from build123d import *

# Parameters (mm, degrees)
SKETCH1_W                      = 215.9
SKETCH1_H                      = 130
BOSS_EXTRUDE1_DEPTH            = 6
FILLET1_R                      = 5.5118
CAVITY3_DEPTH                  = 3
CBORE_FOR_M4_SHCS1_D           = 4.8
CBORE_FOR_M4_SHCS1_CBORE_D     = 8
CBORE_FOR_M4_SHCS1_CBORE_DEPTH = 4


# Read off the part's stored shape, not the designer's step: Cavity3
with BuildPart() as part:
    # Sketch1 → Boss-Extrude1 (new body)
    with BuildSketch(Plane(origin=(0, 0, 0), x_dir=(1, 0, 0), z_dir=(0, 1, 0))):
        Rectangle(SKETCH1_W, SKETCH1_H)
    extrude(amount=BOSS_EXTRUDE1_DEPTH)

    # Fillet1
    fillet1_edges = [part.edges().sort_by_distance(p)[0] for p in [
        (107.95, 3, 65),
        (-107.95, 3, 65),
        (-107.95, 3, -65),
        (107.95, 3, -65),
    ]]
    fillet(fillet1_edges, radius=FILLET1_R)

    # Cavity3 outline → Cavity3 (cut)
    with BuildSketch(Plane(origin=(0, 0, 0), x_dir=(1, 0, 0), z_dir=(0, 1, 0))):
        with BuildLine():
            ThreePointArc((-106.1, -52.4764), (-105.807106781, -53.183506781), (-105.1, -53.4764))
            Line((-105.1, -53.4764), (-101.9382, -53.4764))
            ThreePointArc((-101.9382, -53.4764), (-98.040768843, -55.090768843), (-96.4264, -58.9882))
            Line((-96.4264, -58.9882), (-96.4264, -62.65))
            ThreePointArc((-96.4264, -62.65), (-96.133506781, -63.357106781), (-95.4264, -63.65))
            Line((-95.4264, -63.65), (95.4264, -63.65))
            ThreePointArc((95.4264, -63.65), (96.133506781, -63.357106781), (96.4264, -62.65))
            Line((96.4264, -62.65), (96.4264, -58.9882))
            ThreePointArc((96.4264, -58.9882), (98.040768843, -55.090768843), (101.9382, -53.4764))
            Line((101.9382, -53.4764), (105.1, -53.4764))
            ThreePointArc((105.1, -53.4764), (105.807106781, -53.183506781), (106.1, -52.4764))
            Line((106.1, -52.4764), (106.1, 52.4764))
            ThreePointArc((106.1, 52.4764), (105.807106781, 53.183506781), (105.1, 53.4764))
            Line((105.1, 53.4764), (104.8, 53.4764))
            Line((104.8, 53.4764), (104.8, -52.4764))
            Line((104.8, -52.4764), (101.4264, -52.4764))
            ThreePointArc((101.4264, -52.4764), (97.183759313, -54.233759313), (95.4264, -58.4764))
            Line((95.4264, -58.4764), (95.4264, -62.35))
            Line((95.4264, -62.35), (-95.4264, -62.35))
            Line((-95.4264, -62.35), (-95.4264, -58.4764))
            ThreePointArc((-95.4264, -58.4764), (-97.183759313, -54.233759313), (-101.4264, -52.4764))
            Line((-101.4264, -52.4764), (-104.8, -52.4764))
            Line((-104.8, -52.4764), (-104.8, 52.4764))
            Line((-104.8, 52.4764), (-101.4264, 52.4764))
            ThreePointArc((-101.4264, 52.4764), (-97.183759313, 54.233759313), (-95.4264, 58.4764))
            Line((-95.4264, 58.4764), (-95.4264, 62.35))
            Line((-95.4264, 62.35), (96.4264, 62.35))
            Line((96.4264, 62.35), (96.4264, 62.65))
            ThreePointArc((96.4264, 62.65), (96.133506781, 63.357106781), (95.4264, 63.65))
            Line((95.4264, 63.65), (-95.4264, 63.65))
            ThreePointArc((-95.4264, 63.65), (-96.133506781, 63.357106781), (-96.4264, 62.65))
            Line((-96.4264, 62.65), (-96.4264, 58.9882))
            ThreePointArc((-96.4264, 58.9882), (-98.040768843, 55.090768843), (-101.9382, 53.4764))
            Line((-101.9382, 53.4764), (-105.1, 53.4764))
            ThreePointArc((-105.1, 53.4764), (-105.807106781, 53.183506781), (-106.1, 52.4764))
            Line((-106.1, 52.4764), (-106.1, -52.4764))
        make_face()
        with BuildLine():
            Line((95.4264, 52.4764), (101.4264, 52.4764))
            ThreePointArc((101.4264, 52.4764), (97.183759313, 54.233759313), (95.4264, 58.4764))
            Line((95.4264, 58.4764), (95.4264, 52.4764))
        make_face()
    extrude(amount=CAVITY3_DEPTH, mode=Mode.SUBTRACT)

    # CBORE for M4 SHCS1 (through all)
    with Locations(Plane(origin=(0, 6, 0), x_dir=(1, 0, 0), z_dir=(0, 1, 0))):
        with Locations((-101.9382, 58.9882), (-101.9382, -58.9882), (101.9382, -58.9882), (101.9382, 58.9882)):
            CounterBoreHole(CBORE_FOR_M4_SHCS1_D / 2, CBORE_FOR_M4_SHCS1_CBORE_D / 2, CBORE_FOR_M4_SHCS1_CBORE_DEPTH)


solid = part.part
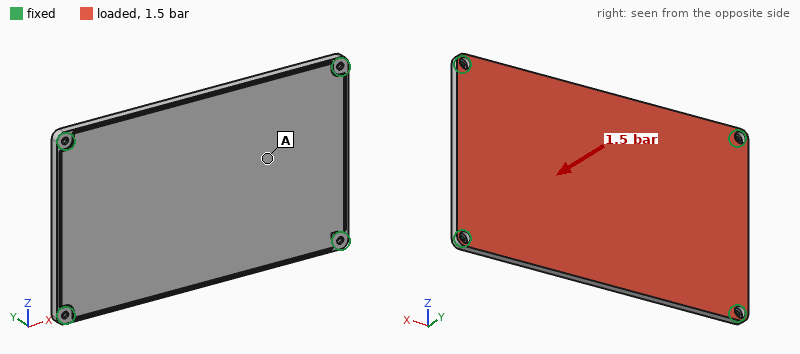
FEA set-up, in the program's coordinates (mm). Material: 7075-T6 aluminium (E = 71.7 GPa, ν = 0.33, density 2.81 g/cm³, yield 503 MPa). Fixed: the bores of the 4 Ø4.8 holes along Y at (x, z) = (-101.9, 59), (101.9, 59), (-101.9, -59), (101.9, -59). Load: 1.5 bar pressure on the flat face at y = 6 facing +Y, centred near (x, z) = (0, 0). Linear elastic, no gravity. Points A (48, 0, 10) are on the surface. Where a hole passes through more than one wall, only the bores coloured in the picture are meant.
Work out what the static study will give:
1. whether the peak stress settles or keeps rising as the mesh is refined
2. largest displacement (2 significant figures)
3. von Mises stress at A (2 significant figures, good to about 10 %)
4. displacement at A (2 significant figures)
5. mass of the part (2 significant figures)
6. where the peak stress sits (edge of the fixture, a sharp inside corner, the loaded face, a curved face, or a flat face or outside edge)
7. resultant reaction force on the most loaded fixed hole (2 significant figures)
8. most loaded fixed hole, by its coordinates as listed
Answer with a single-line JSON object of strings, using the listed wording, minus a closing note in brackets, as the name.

{"whether the peak stress settles or keeps rising as the mesh is refined": "keeps rising", "largest displacement": "1.5 mm", "von Mises stress at A": "46 MPa", "displacement at A": "1.1 mm", "mass of the part": "460 g", "where the peak stress sits": "edge of the fixture", "resultant reaction force on the most loaded fixed hole": "2.5 kN", "most loaded fixed hole, by its coordinates as listed": "(101.9, -59)"}
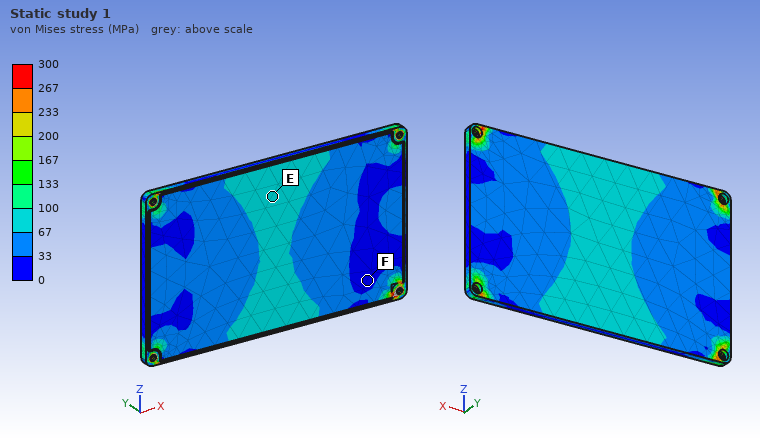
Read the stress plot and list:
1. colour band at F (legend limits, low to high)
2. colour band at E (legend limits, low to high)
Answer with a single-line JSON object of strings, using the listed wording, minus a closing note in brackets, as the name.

{"colour band at F": "0 to 33 MPa", "colour band at E": "67 to 100 MPa"}
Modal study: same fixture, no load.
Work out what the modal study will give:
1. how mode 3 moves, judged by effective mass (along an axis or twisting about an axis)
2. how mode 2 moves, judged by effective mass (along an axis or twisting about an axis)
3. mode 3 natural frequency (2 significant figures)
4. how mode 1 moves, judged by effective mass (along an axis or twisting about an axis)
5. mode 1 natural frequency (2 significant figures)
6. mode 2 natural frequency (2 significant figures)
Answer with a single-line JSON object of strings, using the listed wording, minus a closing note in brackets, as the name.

{"how mode 3 moves, judged by effective mass": "twisting about Z", "how mode 2 moves, judged by effective mass": "twisting about X", "mode 3 natural frequency": "1300 Hz", "how mode 1 moves, judged by effective mass": "along Y", "mode 1 natural frequency": "440 Hz", "mode 2 natural frequency": "900 Hz"}
